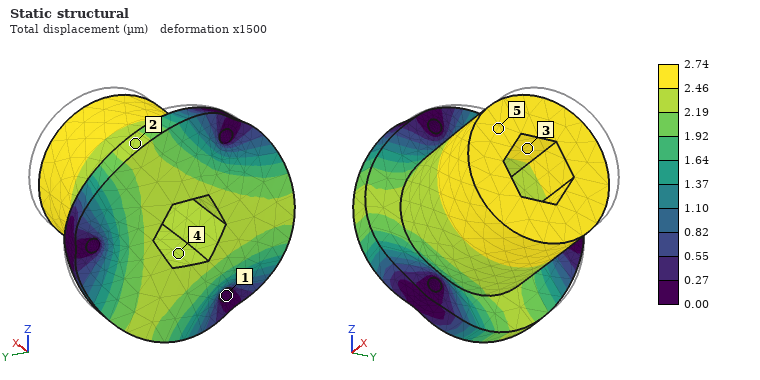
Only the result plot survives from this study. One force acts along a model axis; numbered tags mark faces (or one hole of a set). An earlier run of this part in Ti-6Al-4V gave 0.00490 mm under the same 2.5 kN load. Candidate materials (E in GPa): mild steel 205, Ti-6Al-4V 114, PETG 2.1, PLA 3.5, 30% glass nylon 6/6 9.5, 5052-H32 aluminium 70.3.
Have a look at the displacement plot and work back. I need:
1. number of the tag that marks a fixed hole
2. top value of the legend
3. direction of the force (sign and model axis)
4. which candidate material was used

1
2.74 µm
-X
mild steel
